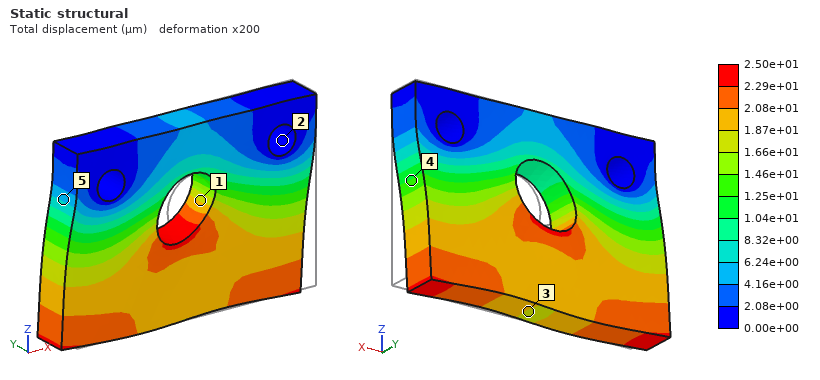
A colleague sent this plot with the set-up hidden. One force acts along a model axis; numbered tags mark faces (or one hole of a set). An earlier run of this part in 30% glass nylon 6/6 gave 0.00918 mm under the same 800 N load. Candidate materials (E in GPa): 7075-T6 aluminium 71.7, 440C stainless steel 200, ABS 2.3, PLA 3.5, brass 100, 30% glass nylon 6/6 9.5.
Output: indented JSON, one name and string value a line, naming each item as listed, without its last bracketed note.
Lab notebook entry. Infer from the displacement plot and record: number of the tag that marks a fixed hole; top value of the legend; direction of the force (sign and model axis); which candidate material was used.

{
  "number of the tag that marks a fixed hole": "2",
  "top value of the legend": "2.50e+01 µm",
  "direction of the force": "-X",
  "which candidate material was used": "PLA"
}
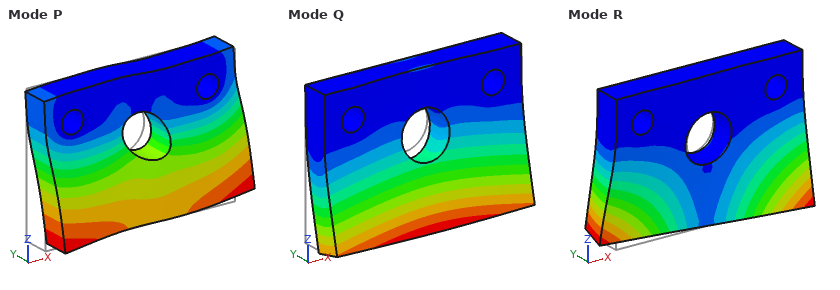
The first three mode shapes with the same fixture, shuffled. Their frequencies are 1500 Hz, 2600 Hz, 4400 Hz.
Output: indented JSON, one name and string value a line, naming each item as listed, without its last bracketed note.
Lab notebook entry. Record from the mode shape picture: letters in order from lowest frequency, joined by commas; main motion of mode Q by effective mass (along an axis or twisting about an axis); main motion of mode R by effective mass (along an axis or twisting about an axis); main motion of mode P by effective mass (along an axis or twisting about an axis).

{
  "letters in order from lowest frequency, joined by commas": "Q, R, P",
  "main motion of mode Q by effective mass": "along Y",
  "main motion of mode R by effective mass": "twisting about Z",
  "main motion of mode P by effective mass": "along X"
}
